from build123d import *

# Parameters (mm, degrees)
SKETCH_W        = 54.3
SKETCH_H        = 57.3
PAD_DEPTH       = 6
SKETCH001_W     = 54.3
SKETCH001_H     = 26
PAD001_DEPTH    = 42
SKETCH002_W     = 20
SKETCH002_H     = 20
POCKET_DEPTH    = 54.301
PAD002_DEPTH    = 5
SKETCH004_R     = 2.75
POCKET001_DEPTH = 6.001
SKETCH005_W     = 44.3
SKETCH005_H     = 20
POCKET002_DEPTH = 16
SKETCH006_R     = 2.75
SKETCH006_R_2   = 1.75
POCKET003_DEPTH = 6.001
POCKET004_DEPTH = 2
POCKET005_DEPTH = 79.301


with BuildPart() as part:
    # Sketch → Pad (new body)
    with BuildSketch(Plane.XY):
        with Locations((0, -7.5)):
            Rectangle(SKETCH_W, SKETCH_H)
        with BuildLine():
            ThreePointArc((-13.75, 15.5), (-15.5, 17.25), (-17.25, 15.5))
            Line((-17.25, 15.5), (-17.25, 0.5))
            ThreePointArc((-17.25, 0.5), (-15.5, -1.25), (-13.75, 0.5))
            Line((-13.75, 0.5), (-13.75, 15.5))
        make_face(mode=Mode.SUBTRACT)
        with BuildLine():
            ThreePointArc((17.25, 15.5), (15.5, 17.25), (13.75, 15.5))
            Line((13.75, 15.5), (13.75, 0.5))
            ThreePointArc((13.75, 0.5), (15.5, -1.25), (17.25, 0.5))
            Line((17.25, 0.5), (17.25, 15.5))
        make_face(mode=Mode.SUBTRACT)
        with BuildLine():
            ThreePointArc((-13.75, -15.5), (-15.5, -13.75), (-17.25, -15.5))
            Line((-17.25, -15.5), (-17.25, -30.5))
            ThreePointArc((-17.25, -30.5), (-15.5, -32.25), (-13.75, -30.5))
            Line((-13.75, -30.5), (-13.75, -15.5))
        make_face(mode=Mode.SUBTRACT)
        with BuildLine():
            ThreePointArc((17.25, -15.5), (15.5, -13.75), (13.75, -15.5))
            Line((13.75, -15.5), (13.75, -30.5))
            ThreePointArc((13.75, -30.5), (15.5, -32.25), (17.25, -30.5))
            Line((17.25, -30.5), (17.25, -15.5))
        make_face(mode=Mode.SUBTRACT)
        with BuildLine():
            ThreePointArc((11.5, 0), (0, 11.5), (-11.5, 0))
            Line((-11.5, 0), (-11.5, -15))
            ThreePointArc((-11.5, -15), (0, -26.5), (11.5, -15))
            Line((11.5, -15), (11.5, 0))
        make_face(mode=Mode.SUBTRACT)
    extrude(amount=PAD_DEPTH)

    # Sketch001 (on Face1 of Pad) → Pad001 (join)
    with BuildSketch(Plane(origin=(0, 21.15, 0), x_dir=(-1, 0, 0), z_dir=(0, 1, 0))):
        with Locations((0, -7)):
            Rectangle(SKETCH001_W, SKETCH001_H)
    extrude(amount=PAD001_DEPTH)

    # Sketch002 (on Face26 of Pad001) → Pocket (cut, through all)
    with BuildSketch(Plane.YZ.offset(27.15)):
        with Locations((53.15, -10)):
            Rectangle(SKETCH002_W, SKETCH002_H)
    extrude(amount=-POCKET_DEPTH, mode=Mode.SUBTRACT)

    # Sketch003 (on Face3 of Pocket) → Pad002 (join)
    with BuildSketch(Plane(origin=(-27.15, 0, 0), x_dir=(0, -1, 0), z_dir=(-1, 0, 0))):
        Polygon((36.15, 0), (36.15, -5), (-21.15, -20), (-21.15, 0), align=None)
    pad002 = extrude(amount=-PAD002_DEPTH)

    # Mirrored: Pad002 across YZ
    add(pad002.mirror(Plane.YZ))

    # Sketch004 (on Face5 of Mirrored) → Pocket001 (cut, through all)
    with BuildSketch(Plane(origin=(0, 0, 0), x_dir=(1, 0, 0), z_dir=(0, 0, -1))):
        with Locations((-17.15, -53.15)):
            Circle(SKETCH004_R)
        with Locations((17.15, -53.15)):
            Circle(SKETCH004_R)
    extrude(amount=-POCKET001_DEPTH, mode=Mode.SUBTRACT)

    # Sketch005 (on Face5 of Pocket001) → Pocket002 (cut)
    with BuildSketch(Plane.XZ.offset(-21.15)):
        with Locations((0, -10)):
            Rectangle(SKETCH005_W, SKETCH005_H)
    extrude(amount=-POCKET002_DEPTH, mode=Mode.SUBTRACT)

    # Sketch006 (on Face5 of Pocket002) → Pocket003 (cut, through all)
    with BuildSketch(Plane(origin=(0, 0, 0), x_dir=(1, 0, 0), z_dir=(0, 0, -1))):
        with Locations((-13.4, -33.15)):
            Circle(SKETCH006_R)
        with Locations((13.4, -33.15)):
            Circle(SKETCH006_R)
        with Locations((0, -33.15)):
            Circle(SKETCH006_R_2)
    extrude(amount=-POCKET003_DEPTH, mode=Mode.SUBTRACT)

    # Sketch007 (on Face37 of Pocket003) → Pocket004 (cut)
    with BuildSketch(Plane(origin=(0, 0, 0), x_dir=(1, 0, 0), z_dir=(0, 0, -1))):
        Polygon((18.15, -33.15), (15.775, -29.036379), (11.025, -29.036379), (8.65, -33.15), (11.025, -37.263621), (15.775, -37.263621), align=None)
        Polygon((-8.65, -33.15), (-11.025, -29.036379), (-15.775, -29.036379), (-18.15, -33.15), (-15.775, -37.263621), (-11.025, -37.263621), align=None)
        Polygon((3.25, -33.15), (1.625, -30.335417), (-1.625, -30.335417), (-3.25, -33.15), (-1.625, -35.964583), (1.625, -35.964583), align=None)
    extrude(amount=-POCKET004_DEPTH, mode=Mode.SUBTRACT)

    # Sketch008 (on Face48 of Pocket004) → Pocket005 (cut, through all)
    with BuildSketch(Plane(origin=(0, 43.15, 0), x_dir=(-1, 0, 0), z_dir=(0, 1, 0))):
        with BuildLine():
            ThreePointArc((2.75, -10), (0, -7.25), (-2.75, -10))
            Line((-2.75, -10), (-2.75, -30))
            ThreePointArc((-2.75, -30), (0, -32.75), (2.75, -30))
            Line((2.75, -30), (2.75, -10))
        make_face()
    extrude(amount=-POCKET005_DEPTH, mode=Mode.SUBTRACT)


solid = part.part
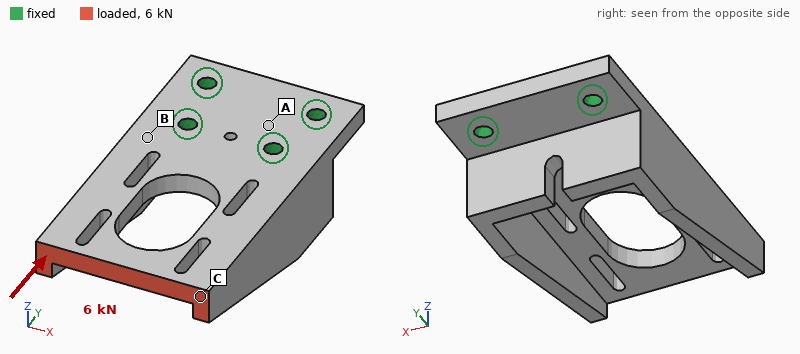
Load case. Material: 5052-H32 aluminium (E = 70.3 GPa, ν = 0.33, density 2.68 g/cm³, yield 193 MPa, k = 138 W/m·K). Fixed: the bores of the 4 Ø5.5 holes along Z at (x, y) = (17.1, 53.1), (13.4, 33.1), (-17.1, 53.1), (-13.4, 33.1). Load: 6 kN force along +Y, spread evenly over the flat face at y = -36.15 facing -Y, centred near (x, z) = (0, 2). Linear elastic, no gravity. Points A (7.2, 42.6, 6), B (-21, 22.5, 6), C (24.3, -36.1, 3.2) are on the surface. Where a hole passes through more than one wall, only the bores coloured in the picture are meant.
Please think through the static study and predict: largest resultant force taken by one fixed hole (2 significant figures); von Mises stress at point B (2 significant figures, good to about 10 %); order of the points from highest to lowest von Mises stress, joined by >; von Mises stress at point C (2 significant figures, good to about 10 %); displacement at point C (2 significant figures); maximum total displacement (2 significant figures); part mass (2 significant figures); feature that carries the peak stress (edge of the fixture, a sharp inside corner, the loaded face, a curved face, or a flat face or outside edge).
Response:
2.0 kN
30 MPa
B > C > A
18 MPa
39 µm
62 µm
110 g
a curved face
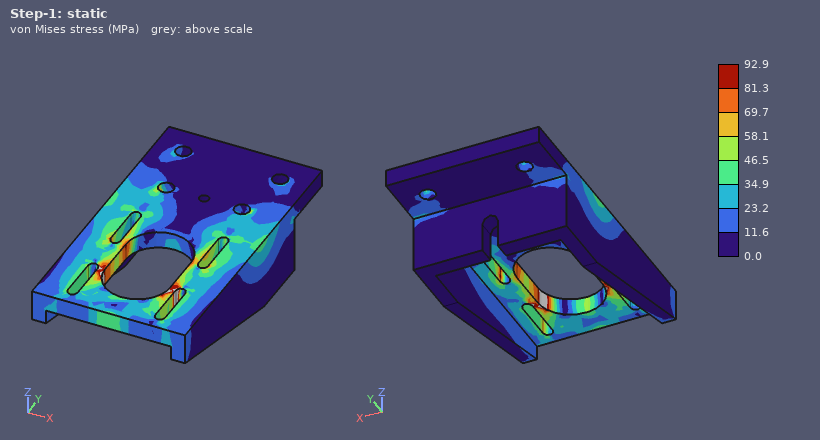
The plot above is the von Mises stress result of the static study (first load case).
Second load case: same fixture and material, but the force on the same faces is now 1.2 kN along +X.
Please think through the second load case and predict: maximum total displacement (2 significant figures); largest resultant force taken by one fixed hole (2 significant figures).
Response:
0.15 mm
1.5 kN
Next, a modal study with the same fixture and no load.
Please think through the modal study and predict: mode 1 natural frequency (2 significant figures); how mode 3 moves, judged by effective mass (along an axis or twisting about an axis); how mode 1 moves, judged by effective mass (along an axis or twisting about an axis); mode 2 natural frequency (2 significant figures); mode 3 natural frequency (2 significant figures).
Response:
2000 Hz
along X
along Z
2600 Hz
3800 Hz
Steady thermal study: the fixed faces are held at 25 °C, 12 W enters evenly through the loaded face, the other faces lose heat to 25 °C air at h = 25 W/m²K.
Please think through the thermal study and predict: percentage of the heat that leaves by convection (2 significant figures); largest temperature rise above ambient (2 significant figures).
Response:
20 %
21 K
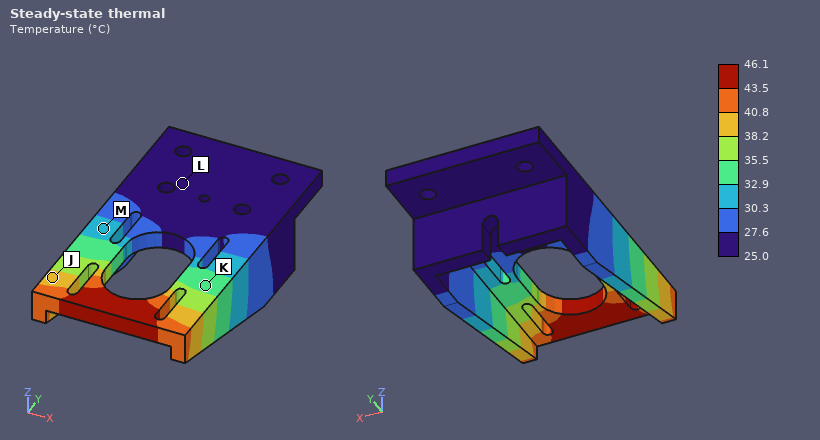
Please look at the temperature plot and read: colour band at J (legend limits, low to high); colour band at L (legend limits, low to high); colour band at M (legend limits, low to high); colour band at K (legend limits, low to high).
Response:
38.2 to 40.8 °C
25.0 to 27.6 °C
30.3 to 32.9 °C
32.9 to 35.5 °C
